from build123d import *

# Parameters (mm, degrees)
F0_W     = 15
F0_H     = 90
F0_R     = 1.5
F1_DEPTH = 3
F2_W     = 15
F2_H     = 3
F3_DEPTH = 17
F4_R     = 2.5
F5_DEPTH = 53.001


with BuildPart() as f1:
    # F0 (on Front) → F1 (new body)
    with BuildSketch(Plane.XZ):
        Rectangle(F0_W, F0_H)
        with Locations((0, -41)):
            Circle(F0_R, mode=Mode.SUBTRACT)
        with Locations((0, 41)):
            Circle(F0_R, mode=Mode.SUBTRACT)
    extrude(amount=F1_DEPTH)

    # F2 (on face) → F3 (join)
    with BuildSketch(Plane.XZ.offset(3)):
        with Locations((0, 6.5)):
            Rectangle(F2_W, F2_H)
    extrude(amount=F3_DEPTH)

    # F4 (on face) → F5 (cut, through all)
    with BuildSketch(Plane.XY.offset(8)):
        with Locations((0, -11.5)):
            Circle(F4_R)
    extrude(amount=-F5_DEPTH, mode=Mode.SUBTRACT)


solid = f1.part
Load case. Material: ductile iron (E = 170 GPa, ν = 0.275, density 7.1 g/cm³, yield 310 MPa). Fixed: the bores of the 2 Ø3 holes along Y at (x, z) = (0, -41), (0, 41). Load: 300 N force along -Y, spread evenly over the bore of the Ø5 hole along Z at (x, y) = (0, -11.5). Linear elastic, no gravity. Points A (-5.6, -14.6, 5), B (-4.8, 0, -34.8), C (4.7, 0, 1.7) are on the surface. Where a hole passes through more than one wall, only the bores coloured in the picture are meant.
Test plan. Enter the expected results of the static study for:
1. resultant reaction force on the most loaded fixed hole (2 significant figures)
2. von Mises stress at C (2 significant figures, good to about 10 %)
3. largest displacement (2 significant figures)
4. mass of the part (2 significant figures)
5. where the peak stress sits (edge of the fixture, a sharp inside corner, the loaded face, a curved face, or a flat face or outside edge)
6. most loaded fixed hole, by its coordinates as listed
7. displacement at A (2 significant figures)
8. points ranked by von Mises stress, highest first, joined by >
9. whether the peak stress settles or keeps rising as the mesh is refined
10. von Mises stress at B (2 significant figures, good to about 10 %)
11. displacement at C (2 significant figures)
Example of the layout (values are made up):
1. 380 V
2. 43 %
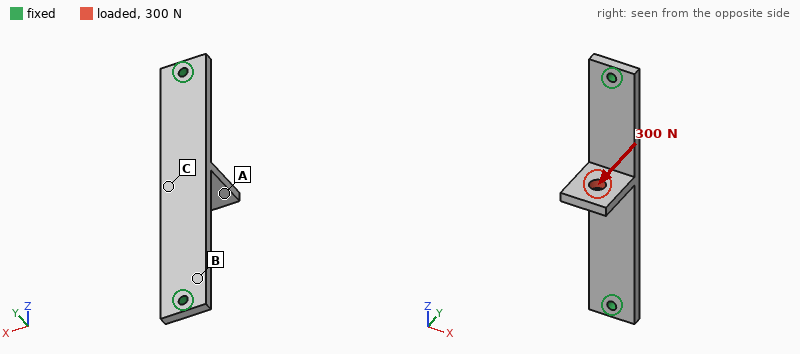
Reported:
1. 190 N
2. 100 MPa
3. 0.14 mm
4. 33 g
5. edge of the fixture
6. (0, 41)
7. 0.14 mm
8. C > B > A
9. keeps rising
10. 76 MPa
11. 0.14 mm
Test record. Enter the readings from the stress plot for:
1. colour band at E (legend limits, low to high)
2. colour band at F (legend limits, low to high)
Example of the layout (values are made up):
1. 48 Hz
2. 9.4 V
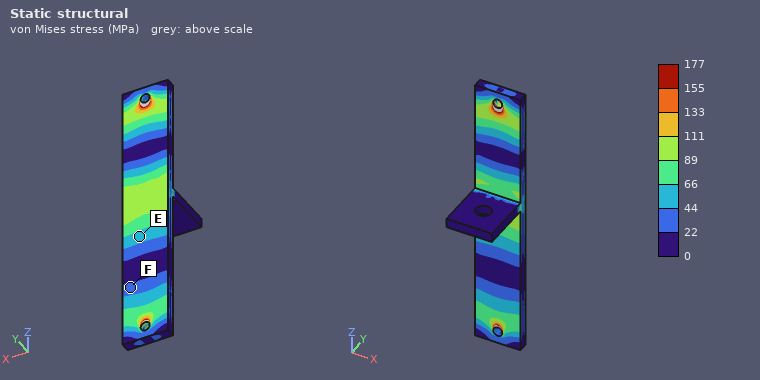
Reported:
1. 44 to 66 MPa
2. 22 to 44 MPa
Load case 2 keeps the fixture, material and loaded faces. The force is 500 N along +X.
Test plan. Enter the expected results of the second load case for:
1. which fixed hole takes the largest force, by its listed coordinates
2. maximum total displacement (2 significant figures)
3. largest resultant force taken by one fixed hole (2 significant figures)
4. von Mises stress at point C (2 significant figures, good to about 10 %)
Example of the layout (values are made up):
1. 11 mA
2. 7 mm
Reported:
1. (0, 41)
2. 0.26 mm
3. 300 N
4. 80 MPa
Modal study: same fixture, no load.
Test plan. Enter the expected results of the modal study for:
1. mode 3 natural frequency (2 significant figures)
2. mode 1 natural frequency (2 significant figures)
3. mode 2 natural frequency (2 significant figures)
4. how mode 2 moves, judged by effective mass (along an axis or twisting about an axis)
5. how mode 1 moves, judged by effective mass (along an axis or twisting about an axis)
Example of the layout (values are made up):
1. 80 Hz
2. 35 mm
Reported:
1. 4500 Hz
2. 1900 Hz
3. 3300 Hz
4. along X
5. along Y
